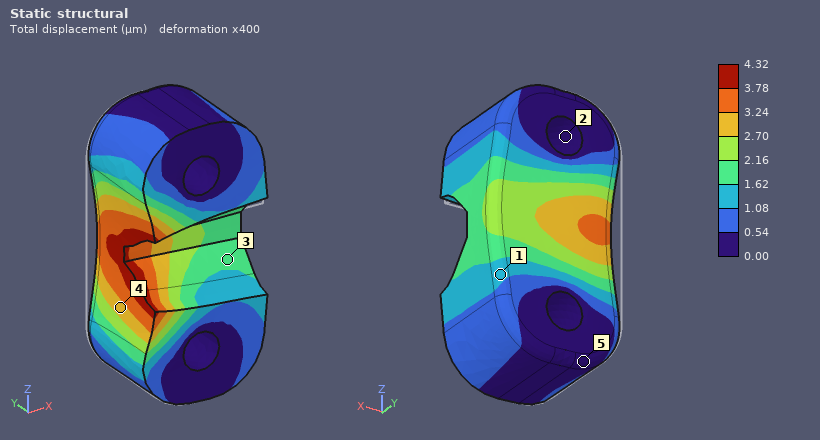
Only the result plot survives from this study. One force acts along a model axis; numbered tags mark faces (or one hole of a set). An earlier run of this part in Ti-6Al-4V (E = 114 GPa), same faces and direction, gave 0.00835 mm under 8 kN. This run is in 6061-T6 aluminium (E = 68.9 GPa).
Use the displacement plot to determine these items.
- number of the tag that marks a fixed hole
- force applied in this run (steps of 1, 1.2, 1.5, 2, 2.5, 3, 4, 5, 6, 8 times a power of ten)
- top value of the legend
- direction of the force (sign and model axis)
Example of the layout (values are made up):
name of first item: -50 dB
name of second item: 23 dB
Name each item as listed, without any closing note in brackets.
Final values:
number of the tag that marks a fixed hole: 2
force applied in this run: 2.5 kN
top value of the legend: 4.32 µm
direction of the force: +X
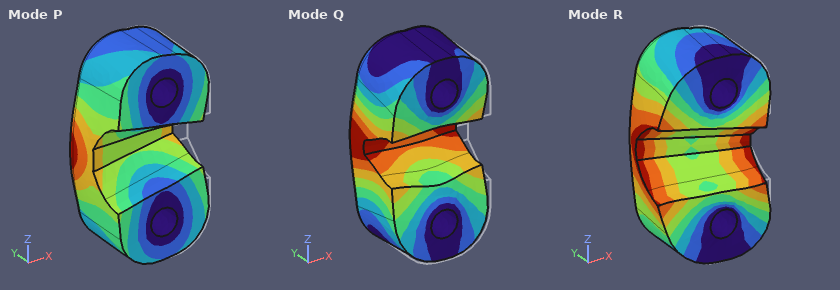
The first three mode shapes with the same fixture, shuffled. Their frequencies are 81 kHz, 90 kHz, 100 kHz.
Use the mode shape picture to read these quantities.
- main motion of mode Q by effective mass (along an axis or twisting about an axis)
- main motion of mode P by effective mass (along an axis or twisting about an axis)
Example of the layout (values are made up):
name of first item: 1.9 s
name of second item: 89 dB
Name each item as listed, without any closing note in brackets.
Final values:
main motion of mode Q by effective mass: along Y
main motion of mode P by effective mass: along X
